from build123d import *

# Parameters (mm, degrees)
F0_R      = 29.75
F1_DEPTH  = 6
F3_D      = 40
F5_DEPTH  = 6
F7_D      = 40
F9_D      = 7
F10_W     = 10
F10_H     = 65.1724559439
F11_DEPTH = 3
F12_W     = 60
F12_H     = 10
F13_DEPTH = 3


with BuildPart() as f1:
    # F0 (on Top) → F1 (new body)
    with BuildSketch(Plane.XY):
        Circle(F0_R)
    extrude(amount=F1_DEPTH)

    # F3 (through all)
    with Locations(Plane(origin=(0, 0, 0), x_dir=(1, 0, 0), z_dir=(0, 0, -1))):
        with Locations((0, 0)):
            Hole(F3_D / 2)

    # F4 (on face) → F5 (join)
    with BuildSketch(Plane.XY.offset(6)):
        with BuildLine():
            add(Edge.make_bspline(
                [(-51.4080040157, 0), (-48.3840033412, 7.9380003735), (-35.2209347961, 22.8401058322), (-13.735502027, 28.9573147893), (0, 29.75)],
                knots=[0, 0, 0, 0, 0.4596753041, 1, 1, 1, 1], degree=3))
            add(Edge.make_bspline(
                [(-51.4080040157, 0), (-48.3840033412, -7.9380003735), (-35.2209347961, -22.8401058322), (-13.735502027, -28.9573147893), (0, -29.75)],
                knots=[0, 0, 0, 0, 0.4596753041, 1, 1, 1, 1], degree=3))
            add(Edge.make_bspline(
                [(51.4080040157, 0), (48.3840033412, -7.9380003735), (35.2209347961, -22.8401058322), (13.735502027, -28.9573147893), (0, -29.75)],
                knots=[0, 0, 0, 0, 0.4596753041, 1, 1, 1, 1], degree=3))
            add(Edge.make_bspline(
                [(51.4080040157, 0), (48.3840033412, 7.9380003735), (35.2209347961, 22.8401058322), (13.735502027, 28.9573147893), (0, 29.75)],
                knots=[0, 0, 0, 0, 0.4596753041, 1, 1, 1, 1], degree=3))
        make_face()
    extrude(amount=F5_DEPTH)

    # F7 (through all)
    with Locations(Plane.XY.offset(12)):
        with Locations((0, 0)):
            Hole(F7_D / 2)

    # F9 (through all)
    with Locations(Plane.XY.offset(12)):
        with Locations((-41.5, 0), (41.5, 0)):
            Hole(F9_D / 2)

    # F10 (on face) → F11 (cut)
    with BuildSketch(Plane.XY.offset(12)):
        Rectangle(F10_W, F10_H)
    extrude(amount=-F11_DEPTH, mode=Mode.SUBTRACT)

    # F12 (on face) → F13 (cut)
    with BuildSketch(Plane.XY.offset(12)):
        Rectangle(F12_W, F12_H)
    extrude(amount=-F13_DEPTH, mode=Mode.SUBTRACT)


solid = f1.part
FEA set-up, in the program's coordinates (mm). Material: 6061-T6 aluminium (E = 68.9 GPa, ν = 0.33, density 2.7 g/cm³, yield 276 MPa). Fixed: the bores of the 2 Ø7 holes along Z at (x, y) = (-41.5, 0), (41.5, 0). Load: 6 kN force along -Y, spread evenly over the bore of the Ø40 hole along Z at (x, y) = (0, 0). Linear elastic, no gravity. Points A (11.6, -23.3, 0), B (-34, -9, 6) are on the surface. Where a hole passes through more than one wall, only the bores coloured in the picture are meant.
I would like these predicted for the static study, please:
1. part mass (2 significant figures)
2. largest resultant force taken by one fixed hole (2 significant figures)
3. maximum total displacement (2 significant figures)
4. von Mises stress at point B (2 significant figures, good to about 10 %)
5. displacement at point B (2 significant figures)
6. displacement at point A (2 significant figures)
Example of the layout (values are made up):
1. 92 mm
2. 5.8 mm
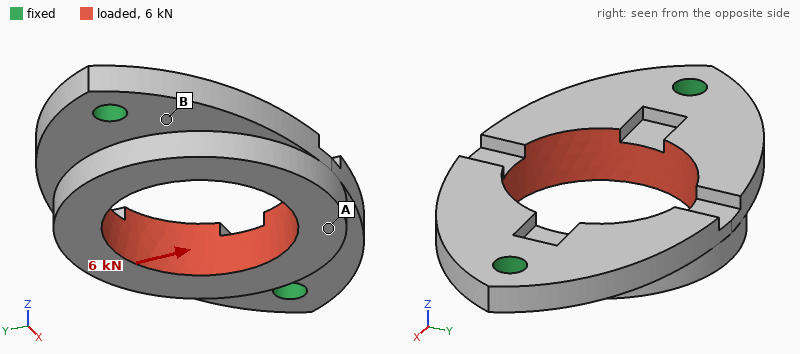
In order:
1. 72 g
2. 3.0 kN
3. 94 µm
4. 46 MPa
5. 17 µm
6. 74 µm
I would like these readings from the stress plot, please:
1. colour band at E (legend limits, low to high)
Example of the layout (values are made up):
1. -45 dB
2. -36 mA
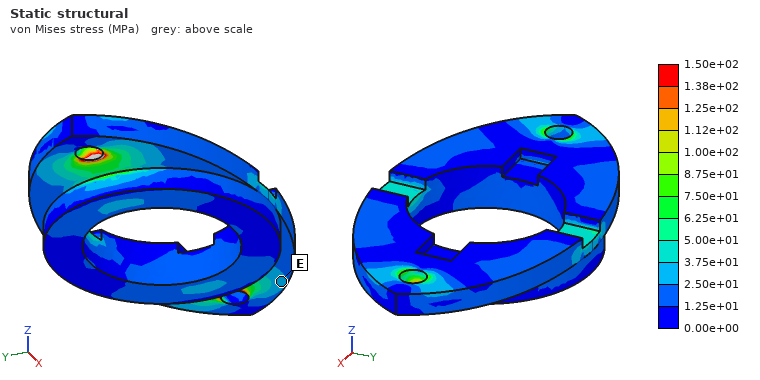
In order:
1. 2.50e+01 to 3.75e+01 MPa
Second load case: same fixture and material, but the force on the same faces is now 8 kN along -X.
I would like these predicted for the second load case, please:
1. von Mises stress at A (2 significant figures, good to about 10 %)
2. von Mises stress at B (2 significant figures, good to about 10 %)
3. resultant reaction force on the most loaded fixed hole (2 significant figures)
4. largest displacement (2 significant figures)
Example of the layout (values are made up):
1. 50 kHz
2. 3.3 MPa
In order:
1. 7.0 MPa
2. 28 MPa
3. 4.0 kN
4. 16 µm
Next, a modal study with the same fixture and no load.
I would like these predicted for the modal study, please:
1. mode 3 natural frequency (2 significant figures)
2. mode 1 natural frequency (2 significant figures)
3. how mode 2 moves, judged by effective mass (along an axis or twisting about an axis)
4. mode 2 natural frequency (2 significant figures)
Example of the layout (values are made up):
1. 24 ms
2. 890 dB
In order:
1. 10000 Hz
2. 3200 Hz
3. along Z
4. 4300 Hz
